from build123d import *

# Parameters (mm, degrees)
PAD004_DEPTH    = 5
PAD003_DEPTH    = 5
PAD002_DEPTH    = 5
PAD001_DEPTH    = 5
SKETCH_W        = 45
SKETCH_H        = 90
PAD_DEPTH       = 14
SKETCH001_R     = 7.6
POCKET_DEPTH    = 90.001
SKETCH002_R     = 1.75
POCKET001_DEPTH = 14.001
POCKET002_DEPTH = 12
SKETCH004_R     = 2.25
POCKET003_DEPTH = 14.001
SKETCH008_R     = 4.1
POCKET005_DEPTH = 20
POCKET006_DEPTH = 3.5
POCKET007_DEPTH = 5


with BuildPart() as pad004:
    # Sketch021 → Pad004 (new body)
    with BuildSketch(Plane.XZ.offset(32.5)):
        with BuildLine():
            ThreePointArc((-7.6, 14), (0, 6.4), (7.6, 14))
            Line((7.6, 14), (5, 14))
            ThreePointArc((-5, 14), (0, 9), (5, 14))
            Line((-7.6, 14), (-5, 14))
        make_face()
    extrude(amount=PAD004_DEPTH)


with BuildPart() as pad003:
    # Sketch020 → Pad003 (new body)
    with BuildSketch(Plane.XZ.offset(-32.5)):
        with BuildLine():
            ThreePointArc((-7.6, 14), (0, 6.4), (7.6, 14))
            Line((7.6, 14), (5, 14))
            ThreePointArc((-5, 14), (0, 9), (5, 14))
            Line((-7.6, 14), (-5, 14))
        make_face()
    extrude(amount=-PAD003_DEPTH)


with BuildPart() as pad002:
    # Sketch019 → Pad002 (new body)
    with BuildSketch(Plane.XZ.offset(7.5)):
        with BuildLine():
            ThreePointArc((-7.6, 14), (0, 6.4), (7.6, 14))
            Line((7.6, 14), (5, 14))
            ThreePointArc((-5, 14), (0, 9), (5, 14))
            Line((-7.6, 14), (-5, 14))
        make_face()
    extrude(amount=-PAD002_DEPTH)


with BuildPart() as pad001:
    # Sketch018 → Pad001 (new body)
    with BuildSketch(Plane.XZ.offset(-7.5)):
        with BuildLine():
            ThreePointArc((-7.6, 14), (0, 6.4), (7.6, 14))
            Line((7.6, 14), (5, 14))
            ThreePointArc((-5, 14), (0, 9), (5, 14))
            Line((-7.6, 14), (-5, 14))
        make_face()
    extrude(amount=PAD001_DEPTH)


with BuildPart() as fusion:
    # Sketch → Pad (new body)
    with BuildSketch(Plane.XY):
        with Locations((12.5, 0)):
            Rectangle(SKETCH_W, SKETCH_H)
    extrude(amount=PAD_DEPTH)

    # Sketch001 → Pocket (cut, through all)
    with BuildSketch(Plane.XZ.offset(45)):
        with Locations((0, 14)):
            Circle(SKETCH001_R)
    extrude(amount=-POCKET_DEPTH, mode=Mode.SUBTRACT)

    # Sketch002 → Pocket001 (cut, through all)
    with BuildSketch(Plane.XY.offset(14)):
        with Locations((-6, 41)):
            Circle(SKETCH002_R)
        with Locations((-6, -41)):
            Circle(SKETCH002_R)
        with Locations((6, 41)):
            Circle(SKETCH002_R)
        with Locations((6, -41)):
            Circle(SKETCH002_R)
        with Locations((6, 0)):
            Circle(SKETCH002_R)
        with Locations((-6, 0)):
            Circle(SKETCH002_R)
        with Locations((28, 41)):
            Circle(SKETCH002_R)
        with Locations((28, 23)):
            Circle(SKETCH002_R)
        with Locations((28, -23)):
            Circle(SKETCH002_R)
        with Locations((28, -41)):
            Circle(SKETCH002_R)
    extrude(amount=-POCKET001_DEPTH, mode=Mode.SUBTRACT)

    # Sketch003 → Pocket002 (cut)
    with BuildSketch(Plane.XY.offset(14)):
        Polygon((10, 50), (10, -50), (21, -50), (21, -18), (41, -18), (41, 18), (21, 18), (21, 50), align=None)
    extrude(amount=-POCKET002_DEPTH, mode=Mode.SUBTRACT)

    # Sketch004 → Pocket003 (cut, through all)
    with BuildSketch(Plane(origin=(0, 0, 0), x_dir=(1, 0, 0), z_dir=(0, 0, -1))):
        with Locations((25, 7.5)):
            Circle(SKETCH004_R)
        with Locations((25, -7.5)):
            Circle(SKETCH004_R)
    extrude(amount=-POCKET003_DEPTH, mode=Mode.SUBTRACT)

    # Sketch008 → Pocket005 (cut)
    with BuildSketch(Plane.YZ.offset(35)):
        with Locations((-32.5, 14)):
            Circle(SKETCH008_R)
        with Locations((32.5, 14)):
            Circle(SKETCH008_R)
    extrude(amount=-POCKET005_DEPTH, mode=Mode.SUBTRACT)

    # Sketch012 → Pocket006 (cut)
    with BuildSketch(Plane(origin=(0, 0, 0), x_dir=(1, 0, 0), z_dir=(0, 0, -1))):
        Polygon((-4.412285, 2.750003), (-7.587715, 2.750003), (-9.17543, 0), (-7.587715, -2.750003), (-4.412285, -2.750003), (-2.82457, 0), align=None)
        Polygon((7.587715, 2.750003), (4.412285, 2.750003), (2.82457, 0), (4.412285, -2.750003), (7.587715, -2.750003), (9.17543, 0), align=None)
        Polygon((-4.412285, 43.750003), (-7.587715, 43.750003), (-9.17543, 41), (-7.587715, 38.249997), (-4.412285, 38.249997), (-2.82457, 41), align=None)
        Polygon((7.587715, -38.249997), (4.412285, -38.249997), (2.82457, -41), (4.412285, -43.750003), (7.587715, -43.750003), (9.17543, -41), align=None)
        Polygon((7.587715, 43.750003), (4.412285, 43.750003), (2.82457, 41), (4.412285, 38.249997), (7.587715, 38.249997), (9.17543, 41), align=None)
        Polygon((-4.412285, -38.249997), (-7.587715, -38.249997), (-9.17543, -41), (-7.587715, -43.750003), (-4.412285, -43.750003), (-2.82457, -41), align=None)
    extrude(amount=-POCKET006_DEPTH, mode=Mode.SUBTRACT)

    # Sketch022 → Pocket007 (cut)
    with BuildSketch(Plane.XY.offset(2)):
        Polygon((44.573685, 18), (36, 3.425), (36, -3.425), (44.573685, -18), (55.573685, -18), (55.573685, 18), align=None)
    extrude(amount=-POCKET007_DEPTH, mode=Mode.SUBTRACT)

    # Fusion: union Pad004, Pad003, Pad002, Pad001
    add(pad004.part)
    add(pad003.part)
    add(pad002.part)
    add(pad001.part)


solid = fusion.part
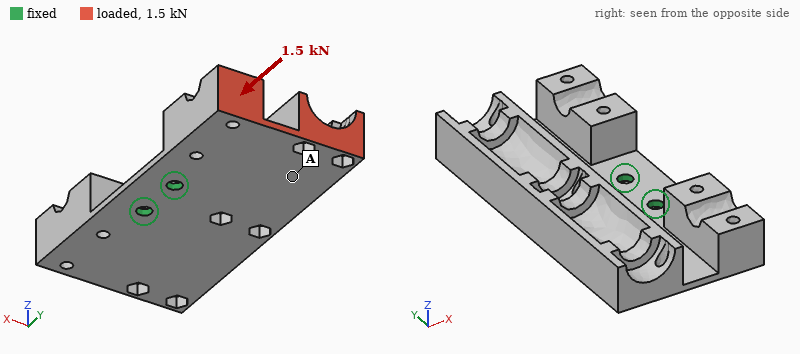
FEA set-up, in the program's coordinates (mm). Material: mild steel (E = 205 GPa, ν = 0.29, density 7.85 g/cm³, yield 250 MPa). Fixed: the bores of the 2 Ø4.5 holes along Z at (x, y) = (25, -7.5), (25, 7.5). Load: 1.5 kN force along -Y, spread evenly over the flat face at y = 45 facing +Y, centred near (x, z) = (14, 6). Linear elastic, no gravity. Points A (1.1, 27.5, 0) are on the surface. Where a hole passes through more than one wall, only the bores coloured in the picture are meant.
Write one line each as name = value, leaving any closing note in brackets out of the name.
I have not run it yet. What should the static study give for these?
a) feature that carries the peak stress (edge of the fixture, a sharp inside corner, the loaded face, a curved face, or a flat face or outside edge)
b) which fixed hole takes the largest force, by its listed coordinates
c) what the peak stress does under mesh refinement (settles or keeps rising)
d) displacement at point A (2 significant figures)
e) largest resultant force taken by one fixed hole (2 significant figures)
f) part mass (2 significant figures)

feature that carries the peak stress = edge of the fixture
which fixed hole takes the largest force, by its listed coordinates = (25, 7.5)
what the peak stress does under mesh refinement = keeps rising
displacement at point A = 0.078 mm
largest resultant force taken by one fixed hole = 1.3 kN
part mass = 230 g
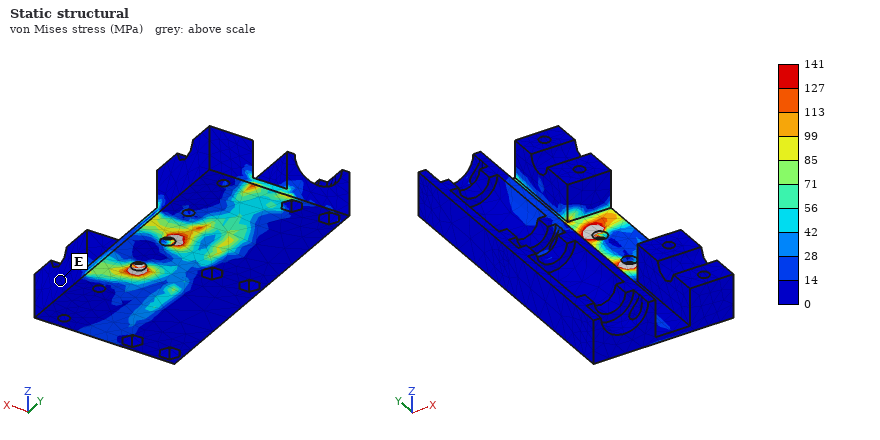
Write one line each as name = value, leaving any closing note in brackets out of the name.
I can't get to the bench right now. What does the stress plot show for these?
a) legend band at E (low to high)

legend band at E = 0 to 14 MPa
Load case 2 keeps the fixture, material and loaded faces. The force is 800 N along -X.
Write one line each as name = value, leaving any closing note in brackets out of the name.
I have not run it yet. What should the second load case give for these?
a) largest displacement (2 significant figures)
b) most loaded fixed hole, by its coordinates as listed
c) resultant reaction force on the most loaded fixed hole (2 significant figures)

largest displacement = 0.15 mm
most loaded fixed hole, by its coordinates as listed = (25, 7.5)
resultant reaction force on the most loaded fixed hole = 2.3 kN
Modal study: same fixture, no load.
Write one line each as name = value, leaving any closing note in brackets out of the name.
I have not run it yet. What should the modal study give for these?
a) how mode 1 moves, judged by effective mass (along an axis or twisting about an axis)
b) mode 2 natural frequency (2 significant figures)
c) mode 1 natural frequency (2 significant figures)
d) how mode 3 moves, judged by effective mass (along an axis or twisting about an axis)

how mode 1 moves, judged by effective mass = along Z
mode 2 natural frequency = 680 Hz
mode 1 natural frequency = 560 Hz
how mode 3 moves, judged by effective mass = along Z
